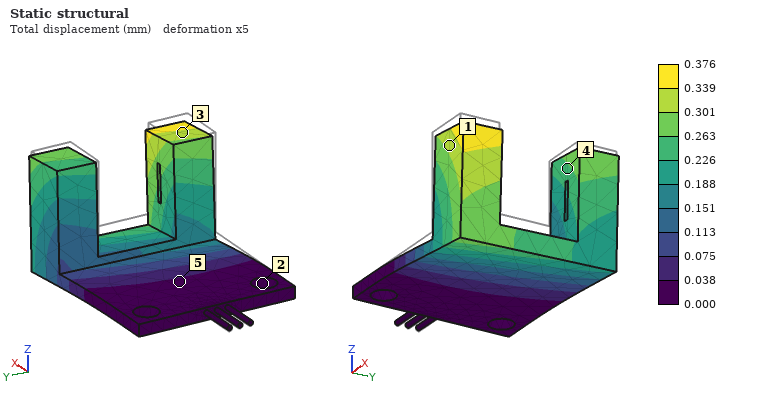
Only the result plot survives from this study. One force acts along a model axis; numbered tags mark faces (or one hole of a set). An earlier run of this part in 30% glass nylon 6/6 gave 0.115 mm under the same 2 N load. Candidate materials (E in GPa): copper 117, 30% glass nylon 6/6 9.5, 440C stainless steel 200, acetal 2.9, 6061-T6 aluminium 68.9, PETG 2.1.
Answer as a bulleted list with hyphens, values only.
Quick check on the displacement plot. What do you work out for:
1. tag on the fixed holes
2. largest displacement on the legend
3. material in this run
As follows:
- 2
- 0.376 mm
- acetal
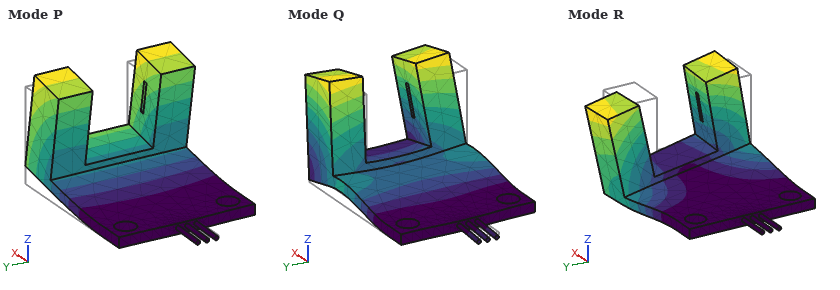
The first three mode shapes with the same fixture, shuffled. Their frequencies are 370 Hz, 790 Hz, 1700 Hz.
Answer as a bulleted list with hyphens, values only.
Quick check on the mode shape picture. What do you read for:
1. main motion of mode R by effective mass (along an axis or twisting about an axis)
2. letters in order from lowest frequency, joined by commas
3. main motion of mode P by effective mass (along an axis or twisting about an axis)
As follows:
- along Y
- P, R, Q
- along Z
